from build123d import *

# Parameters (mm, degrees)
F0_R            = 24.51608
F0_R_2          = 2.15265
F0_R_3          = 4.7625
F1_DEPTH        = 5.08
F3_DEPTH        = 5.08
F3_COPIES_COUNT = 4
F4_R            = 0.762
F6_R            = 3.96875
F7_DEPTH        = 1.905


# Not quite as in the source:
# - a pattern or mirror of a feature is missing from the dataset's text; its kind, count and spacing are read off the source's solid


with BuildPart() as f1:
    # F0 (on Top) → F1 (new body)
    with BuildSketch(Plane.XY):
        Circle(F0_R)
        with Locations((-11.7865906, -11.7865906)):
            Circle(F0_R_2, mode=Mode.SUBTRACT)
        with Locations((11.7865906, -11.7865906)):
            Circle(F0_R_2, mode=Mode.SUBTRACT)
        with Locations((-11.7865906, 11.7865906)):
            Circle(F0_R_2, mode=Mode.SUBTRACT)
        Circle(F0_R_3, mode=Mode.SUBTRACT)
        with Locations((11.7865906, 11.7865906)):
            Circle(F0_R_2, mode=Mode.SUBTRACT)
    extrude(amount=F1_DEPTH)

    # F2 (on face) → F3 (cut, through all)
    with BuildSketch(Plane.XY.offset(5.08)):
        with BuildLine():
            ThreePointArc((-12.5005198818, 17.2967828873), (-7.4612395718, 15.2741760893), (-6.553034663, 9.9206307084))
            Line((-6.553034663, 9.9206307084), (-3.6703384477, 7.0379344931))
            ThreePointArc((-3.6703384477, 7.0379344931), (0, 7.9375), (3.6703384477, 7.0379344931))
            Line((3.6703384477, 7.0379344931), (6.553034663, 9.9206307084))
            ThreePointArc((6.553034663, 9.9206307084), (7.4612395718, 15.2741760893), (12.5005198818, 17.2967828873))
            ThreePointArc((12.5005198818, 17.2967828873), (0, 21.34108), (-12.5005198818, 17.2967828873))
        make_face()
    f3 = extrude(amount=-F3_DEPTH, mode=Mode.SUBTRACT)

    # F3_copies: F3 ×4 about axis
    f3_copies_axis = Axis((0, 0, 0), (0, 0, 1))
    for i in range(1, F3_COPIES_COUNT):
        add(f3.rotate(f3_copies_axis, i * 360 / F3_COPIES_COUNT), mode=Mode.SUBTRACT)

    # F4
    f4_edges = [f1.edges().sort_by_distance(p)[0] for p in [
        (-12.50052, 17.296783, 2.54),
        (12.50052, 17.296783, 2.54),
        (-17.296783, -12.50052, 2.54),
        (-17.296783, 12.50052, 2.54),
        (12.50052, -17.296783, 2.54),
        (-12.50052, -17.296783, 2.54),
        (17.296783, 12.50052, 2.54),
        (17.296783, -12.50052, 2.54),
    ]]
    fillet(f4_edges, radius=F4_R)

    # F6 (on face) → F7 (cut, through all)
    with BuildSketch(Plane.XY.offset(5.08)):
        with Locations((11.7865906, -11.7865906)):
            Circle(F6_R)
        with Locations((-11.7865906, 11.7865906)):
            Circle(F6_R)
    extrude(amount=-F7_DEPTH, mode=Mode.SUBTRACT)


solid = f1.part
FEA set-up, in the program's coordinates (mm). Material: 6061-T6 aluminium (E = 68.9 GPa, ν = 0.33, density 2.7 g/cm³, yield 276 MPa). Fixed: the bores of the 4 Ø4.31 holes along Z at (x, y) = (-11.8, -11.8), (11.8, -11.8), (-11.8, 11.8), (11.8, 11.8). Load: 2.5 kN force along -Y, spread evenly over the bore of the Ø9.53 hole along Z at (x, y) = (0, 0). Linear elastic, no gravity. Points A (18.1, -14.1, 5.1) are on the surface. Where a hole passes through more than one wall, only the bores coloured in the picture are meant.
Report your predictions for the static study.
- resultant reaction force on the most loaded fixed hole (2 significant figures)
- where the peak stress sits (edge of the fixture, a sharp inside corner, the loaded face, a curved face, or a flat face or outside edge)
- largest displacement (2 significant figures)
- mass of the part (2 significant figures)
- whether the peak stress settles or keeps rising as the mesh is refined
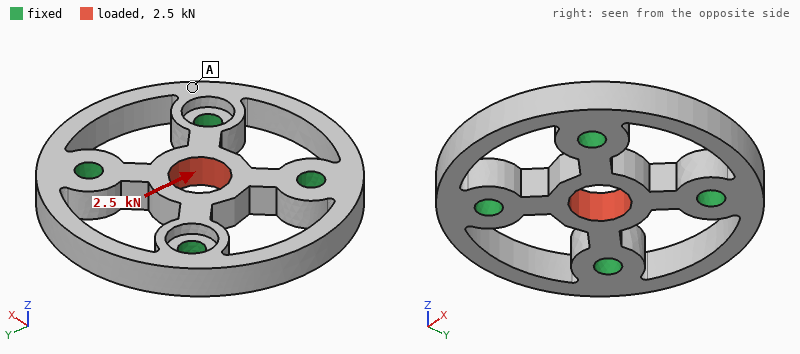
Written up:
760 N
edge of the fixture
12 µm
13 g
keeps rising
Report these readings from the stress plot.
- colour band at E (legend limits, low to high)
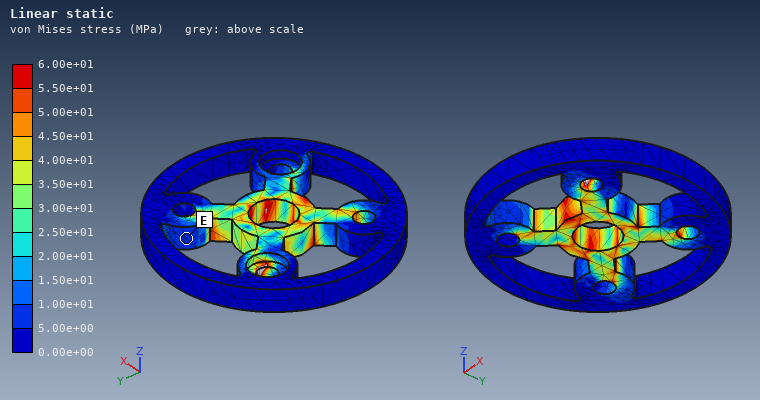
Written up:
5.00e+00 to 1.00e+01 MPa
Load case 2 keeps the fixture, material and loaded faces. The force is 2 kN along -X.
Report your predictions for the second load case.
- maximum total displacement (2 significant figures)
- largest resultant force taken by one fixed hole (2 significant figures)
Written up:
9.2 µm
610 N
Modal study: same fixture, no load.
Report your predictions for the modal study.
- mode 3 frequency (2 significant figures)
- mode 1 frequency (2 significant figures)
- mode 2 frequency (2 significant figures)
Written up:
18 kHz
16 kHz
17 kHz
